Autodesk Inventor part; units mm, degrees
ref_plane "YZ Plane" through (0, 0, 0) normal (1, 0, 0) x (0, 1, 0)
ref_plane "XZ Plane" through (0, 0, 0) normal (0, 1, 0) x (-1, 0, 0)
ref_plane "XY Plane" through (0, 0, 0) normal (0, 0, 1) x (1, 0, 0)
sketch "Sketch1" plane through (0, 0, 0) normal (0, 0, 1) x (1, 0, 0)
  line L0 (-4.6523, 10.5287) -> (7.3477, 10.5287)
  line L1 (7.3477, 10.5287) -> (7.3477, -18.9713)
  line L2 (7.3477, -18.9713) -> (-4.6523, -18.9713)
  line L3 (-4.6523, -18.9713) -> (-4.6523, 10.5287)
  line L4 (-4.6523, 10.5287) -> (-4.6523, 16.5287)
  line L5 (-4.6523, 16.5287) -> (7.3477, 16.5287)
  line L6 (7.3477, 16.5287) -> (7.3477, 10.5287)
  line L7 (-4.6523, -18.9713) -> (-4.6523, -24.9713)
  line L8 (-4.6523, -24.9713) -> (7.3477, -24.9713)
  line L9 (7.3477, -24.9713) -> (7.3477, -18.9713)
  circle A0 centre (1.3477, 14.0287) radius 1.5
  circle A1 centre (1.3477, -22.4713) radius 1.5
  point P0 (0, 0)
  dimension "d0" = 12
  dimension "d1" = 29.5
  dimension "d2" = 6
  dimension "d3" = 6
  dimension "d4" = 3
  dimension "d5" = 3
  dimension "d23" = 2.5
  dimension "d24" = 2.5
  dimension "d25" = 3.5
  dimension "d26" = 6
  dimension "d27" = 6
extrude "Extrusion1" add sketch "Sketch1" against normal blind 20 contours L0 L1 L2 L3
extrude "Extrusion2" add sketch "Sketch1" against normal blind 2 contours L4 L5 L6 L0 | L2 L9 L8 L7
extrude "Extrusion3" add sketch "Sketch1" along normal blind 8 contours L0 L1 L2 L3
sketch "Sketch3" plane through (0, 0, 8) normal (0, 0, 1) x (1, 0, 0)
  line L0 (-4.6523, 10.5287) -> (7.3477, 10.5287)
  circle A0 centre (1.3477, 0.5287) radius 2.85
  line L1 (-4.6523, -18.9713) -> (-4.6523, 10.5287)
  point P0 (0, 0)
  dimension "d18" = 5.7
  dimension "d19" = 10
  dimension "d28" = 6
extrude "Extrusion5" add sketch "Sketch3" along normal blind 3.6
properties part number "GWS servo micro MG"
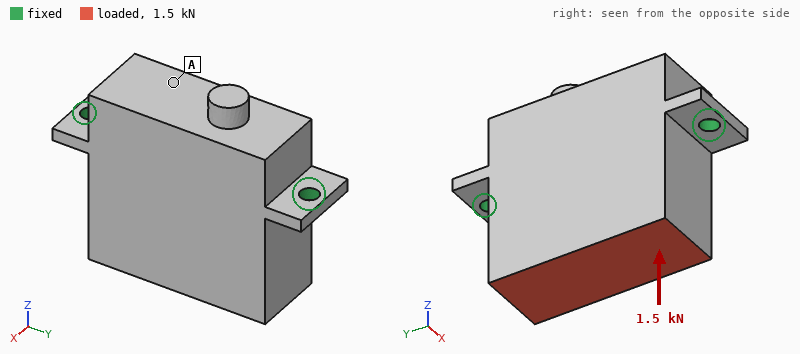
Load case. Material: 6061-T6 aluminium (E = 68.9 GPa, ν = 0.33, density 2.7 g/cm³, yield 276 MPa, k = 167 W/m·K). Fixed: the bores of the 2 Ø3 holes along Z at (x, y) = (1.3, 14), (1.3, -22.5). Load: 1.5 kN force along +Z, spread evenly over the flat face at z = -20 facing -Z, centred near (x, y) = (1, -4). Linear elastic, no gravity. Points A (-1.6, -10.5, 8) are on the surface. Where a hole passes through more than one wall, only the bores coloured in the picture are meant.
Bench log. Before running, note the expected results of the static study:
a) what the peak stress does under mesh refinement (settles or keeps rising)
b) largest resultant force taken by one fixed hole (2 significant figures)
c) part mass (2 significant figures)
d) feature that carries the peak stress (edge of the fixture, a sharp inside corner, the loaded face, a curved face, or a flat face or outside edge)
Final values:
keeps rising
750 N
28 g
edge of the fixture
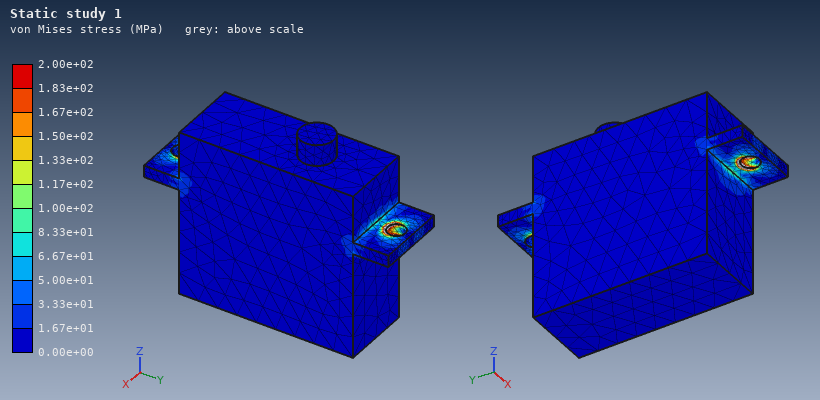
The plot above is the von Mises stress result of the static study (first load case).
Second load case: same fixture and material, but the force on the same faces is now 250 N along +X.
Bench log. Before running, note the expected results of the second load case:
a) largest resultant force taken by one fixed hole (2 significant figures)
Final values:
130 N
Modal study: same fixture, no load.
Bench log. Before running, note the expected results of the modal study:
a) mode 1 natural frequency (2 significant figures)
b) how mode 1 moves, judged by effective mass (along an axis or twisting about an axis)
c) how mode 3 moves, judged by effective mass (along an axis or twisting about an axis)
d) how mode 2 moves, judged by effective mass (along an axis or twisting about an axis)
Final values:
2500 Hz
along X
along Y
along Z
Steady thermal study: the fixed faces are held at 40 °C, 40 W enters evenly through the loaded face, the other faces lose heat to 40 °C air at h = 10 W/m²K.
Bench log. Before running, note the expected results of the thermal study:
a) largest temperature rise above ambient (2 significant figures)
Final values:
38 K
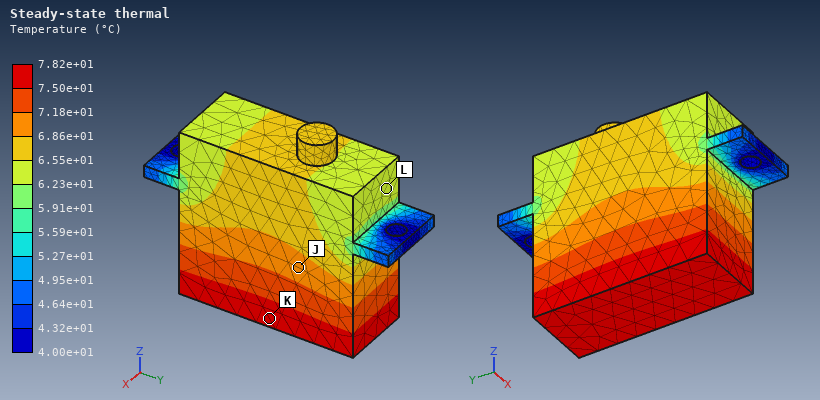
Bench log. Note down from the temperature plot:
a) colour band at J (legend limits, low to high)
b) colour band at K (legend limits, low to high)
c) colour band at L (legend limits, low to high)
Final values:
6.86e+01 to 7.18e+01 °C
7.50e+01 to 7.82e+01 °C
6.23e+01 to 6.55e+01 °C
